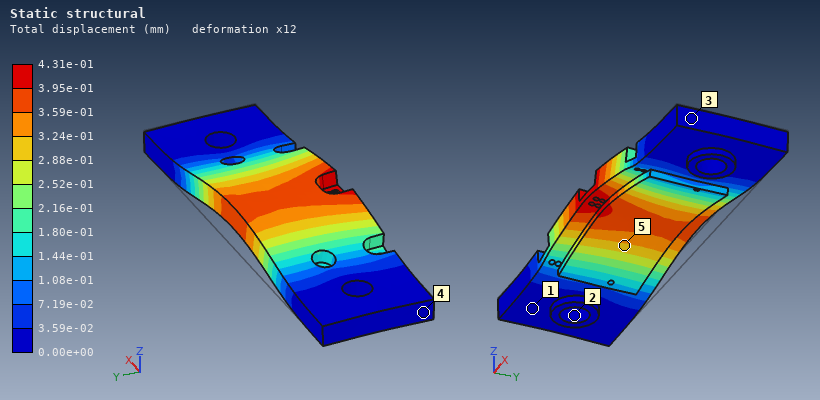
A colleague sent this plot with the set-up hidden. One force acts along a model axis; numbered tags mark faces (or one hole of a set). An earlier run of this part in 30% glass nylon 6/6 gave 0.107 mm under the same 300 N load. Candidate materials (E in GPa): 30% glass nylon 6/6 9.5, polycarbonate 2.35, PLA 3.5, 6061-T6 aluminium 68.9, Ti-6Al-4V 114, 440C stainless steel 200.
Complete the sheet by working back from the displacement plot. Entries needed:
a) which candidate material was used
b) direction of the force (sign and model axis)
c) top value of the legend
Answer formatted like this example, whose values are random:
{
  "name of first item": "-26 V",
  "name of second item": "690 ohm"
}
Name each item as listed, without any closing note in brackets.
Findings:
{
  "which candidate material was used": "polycarbonate",
  "direction of the force": "+Z",
  "top value of the legend": "4.31e-01 mm"
}
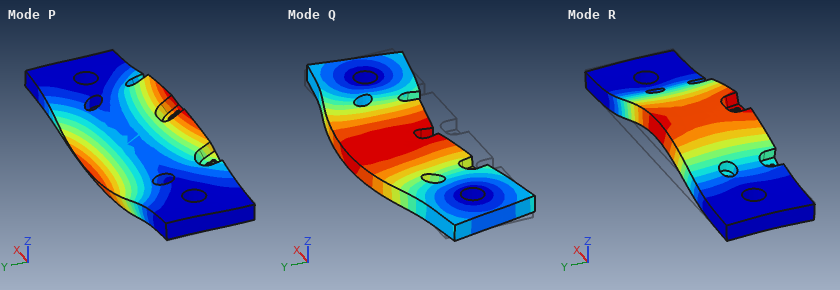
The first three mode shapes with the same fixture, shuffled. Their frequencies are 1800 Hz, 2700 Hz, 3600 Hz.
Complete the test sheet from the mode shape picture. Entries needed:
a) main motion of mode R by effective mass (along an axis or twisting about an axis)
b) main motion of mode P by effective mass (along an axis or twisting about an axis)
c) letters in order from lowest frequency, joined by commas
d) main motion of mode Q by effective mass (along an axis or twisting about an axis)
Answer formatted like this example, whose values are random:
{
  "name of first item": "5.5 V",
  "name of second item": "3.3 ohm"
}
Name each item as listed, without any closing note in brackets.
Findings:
{
  "main motion of mode R by effective mass": "along Z",
  "main motion of mode P by effective mass": "twisting about X",
  "letters in order from lowest frequency, joined by commas": "R, P, Q",
  "main motion of mode Q by effective mass": "along Y"
}
